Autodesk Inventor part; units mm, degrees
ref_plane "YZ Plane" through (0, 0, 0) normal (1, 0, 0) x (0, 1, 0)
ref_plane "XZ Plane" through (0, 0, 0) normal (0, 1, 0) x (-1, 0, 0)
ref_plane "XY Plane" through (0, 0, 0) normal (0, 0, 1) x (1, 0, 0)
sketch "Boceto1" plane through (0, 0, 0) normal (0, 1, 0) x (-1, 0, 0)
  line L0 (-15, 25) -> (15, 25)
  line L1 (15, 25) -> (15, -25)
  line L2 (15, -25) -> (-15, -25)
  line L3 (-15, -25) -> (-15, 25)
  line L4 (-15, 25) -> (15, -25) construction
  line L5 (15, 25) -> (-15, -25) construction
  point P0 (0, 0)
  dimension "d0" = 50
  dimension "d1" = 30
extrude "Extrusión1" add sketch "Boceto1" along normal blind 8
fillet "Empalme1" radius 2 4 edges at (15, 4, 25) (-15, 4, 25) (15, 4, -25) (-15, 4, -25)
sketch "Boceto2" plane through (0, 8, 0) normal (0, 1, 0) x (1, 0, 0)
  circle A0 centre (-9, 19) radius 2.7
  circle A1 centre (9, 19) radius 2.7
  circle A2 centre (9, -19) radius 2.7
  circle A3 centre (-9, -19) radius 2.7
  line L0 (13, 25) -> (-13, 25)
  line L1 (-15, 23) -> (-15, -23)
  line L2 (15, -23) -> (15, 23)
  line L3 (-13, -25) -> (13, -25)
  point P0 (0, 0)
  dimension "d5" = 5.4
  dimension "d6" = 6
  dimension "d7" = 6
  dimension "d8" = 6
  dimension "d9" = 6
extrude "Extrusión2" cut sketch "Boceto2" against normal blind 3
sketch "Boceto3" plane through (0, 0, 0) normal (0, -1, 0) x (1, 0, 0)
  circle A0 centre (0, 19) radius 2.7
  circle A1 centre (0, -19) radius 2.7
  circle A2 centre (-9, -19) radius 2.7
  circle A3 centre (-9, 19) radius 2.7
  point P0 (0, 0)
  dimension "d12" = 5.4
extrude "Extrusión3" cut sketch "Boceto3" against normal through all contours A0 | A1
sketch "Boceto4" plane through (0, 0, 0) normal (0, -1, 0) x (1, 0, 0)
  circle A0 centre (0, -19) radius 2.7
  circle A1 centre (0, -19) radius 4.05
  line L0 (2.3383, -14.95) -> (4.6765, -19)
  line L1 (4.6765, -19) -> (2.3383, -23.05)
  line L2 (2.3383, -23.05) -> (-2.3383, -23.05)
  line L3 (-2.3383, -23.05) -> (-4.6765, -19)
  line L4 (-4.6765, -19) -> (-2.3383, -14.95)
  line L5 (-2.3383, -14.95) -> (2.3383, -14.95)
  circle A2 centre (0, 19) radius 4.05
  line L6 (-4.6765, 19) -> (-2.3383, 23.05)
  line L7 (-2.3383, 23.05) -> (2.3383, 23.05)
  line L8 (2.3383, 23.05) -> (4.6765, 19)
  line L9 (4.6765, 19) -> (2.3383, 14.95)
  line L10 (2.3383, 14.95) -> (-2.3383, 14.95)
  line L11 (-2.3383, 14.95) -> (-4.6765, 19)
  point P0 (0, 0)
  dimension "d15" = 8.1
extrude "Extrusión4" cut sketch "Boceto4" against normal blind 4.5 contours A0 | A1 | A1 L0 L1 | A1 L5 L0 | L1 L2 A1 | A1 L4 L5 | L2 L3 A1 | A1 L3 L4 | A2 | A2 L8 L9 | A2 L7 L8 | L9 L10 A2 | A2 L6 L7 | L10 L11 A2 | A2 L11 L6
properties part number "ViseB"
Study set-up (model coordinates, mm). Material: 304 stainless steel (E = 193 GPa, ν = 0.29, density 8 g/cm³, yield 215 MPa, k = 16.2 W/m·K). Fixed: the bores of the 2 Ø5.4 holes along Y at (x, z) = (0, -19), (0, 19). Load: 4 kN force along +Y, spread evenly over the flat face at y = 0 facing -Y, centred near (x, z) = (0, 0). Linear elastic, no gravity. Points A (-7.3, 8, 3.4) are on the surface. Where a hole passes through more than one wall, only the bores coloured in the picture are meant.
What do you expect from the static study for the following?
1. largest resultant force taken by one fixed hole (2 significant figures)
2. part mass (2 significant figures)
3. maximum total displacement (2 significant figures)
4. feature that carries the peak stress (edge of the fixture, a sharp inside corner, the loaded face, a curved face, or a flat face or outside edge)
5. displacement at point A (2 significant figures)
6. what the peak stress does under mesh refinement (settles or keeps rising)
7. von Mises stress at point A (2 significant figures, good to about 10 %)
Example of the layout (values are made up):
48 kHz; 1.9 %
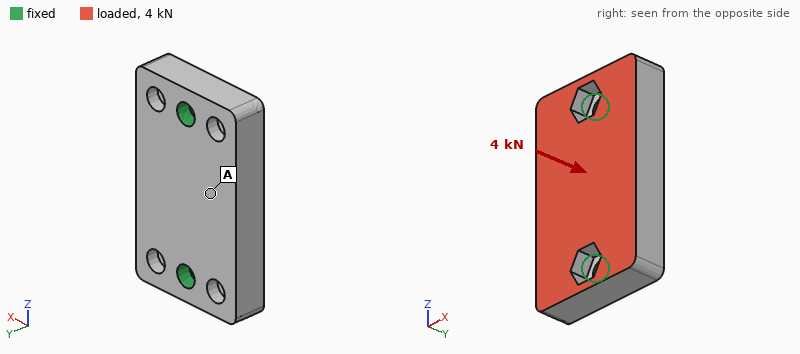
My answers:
2.2 kN; 88 g; 8.4 µm; edge of the fixture; 6.5 µm; keeps rising; 20 MPa
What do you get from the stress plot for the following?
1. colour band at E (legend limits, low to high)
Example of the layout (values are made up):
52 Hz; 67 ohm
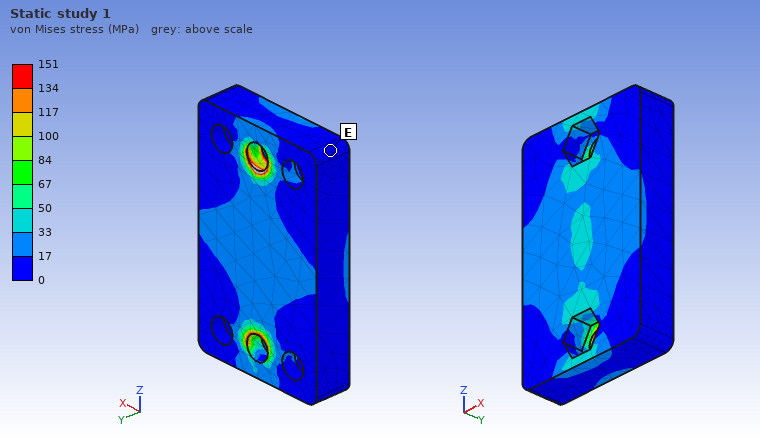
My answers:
0 to 17 MPa
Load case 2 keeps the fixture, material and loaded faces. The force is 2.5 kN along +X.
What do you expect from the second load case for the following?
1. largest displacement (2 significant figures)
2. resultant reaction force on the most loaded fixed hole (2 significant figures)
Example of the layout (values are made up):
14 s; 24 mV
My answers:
13 µm; 1.3 kN
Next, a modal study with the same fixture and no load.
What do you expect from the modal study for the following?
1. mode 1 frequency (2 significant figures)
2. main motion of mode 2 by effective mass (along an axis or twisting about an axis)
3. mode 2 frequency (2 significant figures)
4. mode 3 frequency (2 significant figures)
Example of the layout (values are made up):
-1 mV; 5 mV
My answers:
8600 Hz; along Y; 14 kHz; 19 kHz
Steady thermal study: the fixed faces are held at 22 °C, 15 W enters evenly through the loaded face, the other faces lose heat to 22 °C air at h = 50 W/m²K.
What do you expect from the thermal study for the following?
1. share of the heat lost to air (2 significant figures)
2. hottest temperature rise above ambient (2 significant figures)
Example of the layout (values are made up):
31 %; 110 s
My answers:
21 %; 29 K
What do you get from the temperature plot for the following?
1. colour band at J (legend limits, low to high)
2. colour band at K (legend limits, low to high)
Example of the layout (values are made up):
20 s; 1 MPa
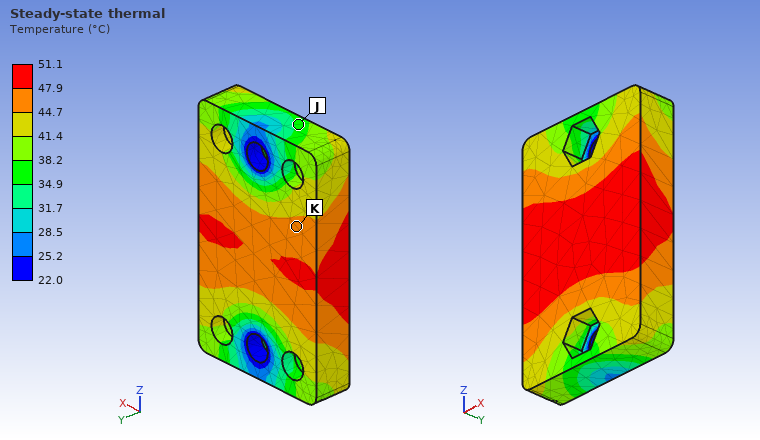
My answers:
34.9 to 38.2 °C; 44.7 to 47.9 °C
